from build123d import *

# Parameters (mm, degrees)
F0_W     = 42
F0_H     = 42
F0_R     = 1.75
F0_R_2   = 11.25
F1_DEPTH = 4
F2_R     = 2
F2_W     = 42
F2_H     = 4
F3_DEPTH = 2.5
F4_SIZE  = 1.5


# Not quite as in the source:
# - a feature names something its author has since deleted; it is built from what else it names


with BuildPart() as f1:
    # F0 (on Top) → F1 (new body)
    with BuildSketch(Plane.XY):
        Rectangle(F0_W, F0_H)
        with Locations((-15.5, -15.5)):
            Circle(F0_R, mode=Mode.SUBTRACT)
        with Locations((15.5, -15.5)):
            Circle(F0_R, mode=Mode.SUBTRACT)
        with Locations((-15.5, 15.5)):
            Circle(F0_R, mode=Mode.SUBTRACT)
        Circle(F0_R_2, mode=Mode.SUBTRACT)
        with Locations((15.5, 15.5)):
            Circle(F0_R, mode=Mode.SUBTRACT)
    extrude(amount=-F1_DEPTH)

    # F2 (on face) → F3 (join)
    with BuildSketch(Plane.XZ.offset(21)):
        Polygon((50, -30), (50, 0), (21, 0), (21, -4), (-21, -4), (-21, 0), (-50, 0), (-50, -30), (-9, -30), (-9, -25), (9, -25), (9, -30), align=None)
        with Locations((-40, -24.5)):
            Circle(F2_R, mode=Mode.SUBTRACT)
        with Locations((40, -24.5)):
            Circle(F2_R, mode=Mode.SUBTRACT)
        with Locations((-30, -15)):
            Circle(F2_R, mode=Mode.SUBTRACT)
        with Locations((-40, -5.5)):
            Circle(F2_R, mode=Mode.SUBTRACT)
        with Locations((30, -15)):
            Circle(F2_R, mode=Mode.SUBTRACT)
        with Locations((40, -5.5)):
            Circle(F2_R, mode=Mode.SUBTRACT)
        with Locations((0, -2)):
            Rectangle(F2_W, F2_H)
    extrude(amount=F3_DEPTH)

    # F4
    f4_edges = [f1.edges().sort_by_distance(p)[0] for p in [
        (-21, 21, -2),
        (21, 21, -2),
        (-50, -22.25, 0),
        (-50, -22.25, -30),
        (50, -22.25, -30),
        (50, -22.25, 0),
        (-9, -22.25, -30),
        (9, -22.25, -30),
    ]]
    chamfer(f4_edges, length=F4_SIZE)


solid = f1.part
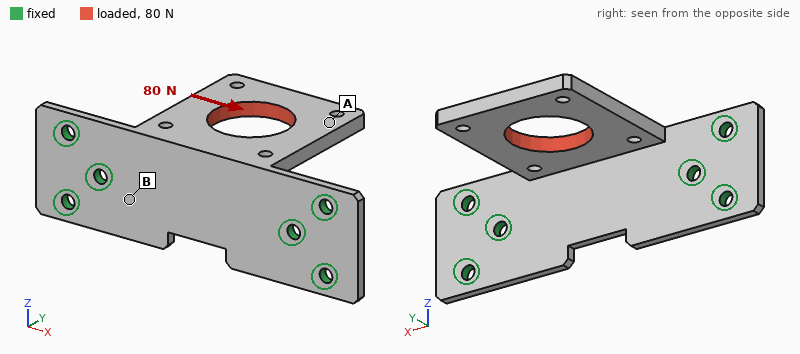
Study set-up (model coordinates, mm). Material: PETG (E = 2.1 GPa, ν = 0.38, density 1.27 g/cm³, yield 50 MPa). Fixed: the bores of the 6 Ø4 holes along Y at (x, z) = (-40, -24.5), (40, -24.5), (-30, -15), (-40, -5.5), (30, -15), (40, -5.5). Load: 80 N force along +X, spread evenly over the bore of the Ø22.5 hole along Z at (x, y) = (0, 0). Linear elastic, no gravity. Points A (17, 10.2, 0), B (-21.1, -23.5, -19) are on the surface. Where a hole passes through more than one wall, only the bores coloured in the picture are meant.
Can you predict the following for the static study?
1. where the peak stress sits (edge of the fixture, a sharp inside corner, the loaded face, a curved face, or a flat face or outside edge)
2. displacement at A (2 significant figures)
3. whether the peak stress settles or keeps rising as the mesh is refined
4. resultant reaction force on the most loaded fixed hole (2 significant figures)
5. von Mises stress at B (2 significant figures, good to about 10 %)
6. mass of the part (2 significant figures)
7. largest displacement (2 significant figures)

edge of the fixture
0.56 mm
keeps rising
36 N
2.4 MPa
16 g
0.75 mm
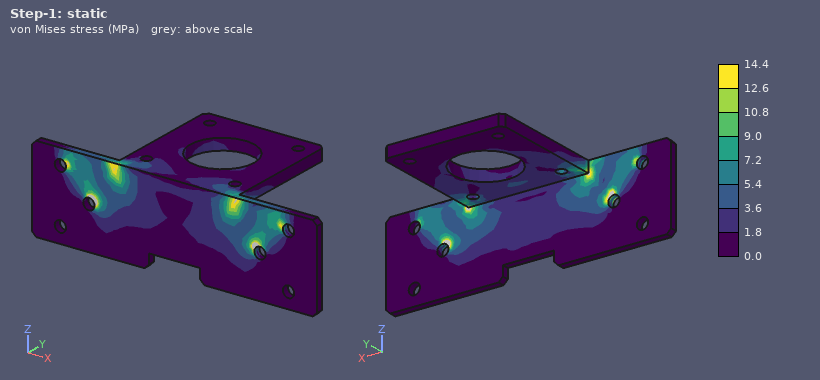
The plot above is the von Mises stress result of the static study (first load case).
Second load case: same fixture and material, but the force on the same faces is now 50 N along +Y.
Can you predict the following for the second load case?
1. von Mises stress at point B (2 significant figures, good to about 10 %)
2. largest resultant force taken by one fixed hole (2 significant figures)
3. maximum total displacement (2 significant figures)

3.2 MPa
22 N
1.2 mm
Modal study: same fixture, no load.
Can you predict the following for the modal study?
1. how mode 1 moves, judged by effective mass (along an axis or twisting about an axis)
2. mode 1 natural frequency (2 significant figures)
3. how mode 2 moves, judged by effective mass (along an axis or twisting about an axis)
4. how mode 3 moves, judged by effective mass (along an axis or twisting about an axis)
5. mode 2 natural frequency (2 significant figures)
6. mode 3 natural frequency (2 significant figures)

along Z
220 Hz
along X
along Y
670 Hz
790 Hz
